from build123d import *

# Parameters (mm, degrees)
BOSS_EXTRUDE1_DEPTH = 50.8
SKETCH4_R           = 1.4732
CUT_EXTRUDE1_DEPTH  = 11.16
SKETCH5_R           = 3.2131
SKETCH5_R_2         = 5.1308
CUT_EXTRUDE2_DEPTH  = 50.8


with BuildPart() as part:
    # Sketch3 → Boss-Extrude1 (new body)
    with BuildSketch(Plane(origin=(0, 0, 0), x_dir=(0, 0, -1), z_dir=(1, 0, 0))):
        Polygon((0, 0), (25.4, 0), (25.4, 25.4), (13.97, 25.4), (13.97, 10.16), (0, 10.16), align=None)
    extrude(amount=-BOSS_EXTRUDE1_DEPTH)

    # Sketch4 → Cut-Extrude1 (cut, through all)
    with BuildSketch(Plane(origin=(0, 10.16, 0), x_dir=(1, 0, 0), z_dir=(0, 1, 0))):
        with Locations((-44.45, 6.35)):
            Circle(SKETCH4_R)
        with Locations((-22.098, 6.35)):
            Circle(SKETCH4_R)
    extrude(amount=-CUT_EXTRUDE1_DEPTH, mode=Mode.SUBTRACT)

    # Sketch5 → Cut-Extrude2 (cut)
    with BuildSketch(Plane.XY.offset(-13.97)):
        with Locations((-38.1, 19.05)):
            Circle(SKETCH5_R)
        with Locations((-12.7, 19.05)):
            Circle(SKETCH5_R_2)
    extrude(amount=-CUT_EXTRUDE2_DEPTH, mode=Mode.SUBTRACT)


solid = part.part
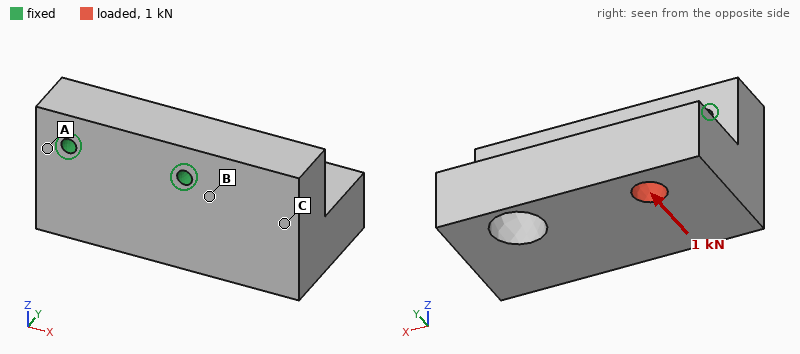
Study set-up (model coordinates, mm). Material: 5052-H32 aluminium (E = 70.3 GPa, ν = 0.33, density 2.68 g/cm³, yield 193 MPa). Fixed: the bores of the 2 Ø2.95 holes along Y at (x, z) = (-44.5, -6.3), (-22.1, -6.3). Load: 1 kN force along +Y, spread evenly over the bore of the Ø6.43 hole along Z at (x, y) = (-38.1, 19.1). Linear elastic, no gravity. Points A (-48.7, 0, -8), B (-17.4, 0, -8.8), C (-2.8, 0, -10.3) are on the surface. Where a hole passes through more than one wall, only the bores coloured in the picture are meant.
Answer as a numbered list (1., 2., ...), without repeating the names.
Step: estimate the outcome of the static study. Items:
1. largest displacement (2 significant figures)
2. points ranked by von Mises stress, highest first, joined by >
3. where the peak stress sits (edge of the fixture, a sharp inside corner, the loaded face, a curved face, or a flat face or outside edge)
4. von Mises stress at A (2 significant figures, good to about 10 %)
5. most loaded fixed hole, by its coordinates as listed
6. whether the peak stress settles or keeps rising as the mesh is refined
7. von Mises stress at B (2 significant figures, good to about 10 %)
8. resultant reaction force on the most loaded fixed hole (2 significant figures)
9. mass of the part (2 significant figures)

1. 18 µm
2. A > B > C
3. edge of the fixture
4. 15 MPa
5. (-44.5, -6.3)
6. keeps rising
7. 7.8 MPa
8. 670 N
9. 55 g
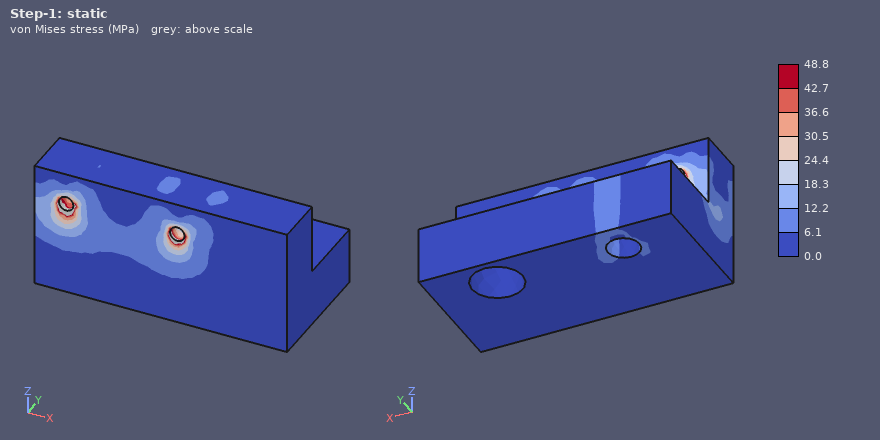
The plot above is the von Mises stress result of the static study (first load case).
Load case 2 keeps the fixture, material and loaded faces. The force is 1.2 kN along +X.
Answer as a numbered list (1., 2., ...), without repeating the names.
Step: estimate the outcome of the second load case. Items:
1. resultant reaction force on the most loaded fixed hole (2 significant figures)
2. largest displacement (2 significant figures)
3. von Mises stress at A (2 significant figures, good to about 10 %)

1. 1.1 kN
2. 13 µm
3. 10 MPa
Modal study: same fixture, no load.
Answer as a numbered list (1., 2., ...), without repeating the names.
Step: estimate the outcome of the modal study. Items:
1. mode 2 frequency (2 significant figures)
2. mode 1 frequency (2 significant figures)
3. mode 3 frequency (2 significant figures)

1. 9800 Hz
2. 6900 Hz
3. 12 kHz
